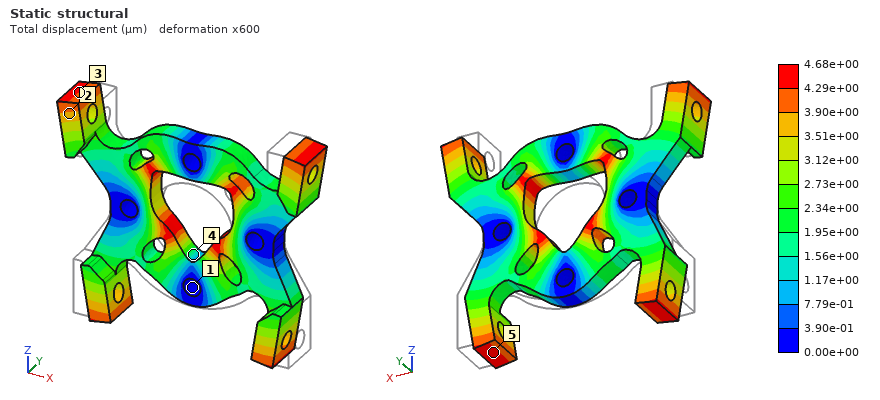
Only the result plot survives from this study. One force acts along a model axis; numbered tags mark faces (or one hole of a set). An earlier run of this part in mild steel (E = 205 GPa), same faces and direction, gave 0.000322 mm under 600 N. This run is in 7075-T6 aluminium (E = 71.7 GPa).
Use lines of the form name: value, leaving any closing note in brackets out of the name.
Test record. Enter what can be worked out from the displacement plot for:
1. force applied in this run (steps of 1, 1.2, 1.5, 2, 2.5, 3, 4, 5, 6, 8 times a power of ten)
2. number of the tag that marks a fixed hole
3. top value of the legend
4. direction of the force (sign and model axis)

force applied in this run: 3 kN
number of the tag that marks a fixed hole: 1
top value of the legend: 4.68e+00 µm
direction of the force: +Z
